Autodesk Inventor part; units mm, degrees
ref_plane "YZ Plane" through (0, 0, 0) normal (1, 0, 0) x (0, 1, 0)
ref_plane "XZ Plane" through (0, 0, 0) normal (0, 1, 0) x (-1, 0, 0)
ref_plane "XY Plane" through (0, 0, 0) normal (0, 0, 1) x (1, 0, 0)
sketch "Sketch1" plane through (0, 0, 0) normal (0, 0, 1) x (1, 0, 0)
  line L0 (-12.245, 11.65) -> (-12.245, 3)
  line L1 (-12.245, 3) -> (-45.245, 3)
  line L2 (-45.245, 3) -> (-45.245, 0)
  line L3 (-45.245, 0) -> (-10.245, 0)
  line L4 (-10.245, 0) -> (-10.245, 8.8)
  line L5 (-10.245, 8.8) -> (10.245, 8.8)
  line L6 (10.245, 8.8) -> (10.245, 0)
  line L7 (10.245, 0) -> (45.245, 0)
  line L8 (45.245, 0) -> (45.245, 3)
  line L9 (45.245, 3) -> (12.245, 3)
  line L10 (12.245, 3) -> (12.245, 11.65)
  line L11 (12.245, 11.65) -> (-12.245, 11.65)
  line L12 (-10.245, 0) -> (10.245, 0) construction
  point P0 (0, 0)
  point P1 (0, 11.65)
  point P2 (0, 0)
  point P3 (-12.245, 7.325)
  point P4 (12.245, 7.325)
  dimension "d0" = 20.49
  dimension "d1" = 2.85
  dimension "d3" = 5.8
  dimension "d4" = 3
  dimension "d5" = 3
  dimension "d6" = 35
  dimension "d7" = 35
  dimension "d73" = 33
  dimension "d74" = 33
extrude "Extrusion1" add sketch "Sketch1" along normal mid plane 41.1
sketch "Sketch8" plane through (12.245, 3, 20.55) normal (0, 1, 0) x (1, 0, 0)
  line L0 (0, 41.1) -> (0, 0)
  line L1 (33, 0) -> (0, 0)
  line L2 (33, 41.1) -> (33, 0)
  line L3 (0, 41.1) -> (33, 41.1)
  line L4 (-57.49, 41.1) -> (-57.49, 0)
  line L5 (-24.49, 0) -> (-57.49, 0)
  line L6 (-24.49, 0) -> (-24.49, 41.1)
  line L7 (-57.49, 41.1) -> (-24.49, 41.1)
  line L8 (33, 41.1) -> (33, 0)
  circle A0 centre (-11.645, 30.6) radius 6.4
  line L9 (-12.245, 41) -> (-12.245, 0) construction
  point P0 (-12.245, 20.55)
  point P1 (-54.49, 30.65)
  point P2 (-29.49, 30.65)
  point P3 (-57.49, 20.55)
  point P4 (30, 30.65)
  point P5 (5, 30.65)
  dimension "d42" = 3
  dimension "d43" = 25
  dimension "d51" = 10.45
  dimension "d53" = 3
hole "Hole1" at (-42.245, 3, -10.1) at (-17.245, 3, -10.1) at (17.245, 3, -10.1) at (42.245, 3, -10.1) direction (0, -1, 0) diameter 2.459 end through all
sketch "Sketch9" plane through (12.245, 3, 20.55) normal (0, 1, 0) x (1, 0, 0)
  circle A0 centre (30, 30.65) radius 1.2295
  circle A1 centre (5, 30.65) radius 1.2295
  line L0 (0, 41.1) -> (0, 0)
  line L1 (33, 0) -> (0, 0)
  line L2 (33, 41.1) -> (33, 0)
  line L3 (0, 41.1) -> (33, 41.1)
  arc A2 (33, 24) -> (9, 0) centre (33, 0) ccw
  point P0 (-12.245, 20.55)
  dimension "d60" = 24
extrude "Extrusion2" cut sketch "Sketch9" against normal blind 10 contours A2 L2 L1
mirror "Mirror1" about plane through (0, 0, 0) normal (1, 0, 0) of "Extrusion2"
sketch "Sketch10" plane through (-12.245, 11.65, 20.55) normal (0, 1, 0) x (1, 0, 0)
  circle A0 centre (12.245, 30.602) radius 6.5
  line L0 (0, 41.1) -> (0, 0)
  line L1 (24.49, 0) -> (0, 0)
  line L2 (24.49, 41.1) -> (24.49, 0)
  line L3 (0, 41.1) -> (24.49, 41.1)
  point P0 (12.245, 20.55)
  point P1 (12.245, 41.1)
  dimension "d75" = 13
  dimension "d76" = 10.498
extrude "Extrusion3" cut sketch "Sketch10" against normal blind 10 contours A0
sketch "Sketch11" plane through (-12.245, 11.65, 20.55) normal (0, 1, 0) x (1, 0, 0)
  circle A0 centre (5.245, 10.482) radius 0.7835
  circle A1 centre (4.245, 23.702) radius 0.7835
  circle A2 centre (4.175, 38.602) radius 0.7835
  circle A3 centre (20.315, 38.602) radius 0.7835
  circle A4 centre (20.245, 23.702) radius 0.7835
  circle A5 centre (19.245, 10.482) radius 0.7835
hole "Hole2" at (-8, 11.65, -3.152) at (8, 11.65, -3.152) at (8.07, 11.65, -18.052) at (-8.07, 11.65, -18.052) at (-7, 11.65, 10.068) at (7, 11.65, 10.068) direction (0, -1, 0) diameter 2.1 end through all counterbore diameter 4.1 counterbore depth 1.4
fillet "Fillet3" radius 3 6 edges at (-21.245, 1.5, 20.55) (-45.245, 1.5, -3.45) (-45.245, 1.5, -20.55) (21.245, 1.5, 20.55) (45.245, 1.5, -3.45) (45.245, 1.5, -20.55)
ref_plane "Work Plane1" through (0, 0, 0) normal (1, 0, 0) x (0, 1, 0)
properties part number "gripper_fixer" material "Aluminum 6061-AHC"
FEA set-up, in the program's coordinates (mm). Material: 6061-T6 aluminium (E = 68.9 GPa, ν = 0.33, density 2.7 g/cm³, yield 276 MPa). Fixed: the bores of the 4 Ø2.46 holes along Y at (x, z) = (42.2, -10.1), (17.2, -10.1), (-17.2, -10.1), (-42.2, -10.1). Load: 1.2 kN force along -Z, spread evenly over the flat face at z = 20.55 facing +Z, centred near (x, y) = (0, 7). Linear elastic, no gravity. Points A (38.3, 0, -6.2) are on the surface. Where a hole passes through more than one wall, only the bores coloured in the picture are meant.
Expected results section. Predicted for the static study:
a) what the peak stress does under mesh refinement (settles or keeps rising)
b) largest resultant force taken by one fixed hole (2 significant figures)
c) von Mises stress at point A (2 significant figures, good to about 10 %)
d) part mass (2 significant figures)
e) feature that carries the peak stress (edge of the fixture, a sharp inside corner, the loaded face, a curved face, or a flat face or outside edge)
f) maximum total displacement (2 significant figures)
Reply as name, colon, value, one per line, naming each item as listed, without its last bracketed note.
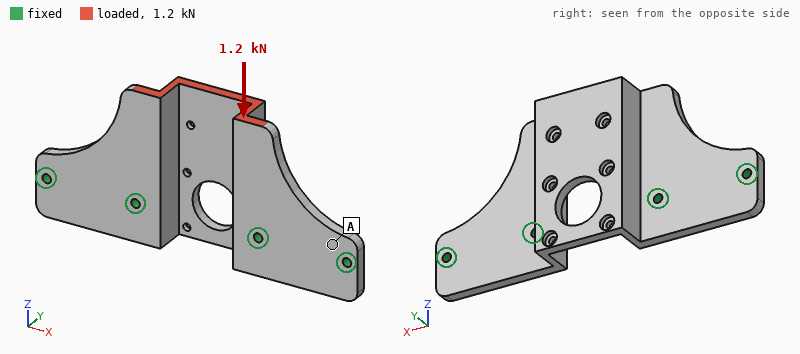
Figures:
what the peak stress does under mesh refinement: keeps rising
largest resultant force taken by one fixed hole: 720 N
von Mises stress at point A: 19 MPa
part mass: 25 g
feature that carries the peak stress: edge of the fixture
maximum total displacement: 0.13 mm
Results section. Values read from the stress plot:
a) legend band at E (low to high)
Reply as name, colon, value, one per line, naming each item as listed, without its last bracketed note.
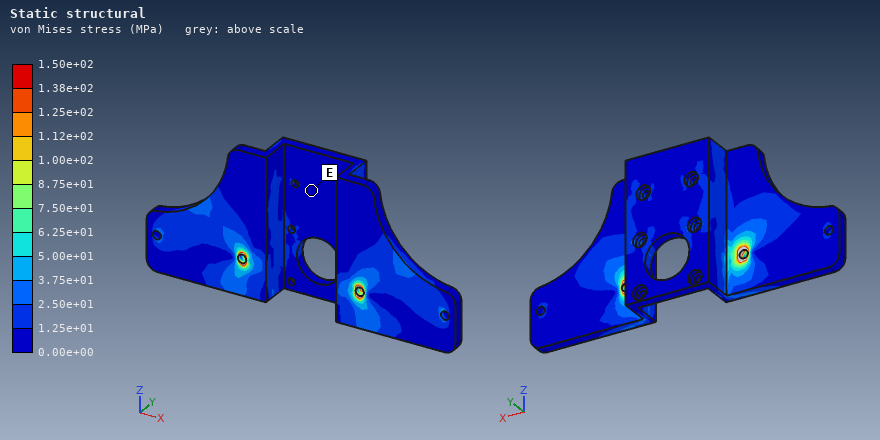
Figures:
legend band at E: 0.00e+00 to 1.25e+01 MPa
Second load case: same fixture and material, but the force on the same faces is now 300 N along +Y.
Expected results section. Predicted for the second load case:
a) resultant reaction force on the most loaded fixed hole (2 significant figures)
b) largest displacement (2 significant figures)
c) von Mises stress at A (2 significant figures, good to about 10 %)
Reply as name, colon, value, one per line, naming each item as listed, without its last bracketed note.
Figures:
resultant reaction force on the most loaded fixed hole: 190 N
largest displacement: 0.21 mm
von Mises stress at A: 28 MPa
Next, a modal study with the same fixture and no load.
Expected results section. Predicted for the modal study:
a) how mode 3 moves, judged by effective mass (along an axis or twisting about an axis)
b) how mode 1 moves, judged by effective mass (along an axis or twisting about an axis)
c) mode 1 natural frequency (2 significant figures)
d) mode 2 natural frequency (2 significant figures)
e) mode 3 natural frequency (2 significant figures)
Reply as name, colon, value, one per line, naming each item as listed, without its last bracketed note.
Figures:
how mode 3 moves, judged by effective mass: along X
how mode 1 moves, judged by effective mass: along Y
mode 1 natural frequency: 2900 Hz
mode 2 natural frequency: 6700 Hz
mode 3 natural frequency: 9500 Hz
